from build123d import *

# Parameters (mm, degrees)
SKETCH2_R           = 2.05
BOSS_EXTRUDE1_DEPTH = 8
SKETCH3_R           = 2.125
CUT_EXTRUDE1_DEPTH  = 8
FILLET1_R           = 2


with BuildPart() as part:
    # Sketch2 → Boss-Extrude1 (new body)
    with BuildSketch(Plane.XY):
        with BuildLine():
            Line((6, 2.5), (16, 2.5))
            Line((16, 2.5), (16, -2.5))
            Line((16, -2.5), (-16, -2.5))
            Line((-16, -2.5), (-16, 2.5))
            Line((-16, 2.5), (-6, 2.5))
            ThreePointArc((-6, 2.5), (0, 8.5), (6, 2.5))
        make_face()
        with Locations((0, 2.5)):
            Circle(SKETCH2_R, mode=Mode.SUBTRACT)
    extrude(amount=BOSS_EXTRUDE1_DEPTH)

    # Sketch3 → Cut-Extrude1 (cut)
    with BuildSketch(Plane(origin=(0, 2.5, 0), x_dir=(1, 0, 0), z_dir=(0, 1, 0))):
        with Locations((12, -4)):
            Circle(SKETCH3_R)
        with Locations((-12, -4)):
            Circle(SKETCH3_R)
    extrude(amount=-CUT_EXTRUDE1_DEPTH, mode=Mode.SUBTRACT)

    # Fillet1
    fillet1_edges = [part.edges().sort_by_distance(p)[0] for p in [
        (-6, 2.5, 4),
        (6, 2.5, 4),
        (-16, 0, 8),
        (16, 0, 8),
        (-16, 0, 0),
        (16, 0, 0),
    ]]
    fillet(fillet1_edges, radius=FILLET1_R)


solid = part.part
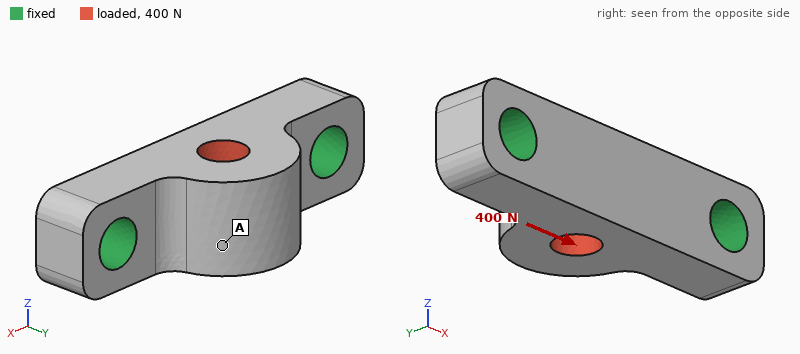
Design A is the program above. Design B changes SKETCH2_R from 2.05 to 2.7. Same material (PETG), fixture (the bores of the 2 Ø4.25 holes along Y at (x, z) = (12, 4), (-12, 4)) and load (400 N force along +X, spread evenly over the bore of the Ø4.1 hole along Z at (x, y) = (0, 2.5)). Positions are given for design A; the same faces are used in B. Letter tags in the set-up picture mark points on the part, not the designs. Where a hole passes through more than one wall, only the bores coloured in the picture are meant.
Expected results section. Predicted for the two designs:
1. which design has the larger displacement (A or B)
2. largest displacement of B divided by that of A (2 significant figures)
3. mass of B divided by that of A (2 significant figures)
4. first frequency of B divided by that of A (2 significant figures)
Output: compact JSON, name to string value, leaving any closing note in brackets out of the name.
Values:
{"which design has the larger displacement": "B", "largest displacement of B divided by that of A": "1.2", "mass of B divided by that of A": "0.95", "first frequency of B divided by that of A": "1.0"}
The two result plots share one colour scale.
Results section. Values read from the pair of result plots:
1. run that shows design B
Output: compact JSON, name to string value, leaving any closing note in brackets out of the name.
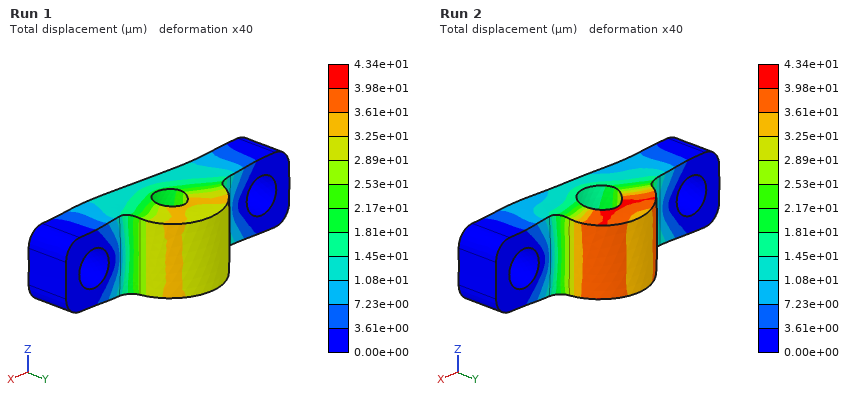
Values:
{"run that shows design B": "Run 2"}
